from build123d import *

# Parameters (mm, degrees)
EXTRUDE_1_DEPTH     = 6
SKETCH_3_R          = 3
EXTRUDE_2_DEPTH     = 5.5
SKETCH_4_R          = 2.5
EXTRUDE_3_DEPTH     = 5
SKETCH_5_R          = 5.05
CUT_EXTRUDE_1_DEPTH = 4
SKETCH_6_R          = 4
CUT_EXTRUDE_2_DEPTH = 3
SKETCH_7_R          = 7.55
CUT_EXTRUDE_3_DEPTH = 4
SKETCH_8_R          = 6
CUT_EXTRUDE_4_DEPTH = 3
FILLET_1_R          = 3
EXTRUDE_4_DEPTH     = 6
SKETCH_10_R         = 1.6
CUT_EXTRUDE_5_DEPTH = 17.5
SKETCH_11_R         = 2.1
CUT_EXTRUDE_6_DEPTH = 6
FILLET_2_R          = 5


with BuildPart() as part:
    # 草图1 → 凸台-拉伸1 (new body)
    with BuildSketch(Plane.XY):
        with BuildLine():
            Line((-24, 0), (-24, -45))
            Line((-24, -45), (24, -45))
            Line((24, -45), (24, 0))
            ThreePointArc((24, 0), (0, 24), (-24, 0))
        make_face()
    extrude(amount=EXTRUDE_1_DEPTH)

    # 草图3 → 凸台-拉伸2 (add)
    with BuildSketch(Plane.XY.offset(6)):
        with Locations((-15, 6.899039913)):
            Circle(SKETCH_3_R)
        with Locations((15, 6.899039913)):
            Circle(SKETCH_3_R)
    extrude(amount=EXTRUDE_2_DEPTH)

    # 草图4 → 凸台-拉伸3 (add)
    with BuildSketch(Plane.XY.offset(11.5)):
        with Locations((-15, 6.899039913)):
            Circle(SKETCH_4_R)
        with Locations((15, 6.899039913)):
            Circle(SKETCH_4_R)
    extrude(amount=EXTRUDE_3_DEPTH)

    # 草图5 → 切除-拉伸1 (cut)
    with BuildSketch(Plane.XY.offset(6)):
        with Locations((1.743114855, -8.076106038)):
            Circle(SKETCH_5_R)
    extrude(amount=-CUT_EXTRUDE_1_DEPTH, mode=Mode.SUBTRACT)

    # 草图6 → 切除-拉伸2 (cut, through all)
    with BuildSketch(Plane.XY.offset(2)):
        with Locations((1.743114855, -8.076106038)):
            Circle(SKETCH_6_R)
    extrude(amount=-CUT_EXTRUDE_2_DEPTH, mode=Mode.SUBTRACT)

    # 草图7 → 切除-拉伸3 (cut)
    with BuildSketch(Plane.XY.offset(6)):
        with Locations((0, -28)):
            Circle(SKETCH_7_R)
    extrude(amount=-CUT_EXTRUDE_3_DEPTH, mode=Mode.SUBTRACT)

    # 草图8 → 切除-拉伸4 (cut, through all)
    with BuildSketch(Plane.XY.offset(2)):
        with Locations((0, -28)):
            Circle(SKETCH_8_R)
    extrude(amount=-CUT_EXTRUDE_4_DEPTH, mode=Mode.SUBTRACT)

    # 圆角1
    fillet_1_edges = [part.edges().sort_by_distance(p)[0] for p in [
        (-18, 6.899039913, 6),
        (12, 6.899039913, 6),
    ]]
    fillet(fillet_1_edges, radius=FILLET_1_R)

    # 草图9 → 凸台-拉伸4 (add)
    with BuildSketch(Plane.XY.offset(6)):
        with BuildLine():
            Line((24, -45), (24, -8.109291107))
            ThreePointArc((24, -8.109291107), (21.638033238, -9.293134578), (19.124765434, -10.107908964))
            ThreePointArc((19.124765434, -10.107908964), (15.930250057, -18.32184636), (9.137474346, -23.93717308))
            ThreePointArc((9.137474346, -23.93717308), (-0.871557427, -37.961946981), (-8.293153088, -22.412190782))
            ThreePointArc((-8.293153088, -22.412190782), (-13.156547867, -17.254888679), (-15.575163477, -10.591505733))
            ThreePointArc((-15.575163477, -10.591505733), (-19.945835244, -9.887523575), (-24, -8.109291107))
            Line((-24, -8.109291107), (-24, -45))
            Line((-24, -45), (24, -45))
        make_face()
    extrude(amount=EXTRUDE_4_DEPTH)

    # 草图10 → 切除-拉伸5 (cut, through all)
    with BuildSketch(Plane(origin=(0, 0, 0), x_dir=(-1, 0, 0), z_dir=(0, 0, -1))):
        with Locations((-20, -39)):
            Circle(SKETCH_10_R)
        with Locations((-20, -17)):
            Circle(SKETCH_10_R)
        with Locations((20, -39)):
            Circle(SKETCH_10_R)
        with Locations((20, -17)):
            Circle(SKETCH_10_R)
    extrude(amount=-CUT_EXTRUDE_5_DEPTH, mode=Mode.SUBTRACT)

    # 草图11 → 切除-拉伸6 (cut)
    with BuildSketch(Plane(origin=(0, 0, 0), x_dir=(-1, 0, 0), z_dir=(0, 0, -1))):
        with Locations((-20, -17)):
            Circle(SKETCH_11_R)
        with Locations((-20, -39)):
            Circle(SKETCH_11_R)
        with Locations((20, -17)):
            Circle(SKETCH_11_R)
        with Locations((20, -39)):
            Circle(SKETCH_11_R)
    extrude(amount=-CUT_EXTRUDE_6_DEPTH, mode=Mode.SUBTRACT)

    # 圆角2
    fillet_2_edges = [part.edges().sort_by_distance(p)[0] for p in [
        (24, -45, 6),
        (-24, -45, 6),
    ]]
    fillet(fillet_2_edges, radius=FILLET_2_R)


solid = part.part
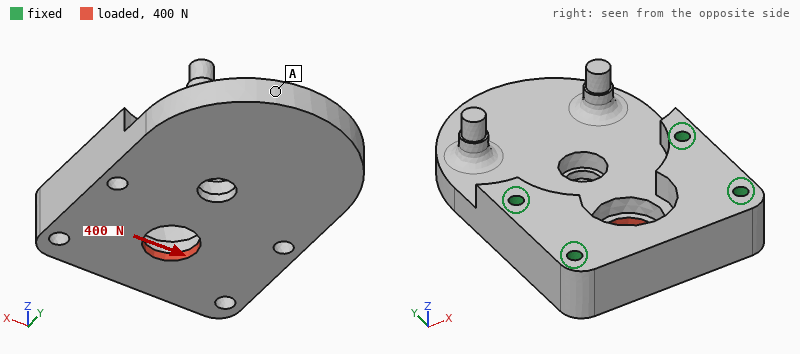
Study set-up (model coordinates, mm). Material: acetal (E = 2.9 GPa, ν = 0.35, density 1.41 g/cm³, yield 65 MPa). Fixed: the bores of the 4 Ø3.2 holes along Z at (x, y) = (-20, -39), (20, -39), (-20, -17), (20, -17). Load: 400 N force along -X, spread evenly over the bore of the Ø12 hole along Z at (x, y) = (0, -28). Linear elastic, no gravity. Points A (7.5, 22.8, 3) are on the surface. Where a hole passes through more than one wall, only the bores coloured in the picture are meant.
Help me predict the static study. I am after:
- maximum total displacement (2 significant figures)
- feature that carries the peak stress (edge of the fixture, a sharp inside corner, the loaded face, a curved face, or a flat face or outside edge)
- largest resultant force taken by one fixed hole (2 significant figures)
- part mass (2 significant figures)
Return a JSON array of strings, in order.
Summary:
["29 µm", "edge of the fixture", "120 N", "33 g"]
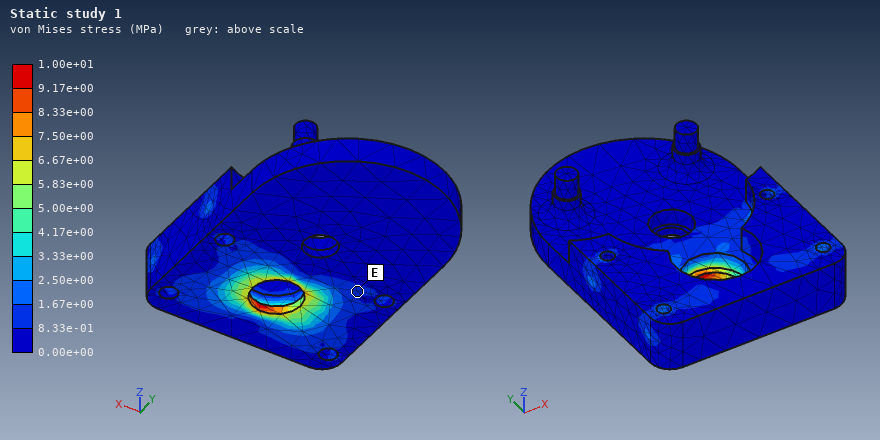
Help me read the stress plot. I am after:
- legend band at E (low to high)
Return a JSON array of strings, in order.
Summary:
["8.33e-01 to 1.67e+00 MPa"]
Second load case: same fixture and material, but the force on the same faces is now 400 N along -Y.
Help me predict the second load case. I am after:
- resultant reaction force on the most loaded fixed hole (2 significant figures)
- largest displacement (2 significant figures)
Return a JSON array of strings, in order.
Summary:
["140 N", "47 µm"]
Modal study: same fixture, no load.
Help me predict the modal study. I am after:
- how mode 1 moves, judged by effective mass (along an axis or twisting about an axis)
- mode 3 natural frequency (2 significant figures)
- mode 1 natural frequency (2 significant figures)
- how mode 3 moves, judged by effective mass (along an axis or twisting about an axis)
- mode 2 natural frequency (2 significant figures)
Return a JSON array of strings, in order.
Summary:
["along Z", "3400 Hz", "890 Hz", "along X", "2300 Hz"]
